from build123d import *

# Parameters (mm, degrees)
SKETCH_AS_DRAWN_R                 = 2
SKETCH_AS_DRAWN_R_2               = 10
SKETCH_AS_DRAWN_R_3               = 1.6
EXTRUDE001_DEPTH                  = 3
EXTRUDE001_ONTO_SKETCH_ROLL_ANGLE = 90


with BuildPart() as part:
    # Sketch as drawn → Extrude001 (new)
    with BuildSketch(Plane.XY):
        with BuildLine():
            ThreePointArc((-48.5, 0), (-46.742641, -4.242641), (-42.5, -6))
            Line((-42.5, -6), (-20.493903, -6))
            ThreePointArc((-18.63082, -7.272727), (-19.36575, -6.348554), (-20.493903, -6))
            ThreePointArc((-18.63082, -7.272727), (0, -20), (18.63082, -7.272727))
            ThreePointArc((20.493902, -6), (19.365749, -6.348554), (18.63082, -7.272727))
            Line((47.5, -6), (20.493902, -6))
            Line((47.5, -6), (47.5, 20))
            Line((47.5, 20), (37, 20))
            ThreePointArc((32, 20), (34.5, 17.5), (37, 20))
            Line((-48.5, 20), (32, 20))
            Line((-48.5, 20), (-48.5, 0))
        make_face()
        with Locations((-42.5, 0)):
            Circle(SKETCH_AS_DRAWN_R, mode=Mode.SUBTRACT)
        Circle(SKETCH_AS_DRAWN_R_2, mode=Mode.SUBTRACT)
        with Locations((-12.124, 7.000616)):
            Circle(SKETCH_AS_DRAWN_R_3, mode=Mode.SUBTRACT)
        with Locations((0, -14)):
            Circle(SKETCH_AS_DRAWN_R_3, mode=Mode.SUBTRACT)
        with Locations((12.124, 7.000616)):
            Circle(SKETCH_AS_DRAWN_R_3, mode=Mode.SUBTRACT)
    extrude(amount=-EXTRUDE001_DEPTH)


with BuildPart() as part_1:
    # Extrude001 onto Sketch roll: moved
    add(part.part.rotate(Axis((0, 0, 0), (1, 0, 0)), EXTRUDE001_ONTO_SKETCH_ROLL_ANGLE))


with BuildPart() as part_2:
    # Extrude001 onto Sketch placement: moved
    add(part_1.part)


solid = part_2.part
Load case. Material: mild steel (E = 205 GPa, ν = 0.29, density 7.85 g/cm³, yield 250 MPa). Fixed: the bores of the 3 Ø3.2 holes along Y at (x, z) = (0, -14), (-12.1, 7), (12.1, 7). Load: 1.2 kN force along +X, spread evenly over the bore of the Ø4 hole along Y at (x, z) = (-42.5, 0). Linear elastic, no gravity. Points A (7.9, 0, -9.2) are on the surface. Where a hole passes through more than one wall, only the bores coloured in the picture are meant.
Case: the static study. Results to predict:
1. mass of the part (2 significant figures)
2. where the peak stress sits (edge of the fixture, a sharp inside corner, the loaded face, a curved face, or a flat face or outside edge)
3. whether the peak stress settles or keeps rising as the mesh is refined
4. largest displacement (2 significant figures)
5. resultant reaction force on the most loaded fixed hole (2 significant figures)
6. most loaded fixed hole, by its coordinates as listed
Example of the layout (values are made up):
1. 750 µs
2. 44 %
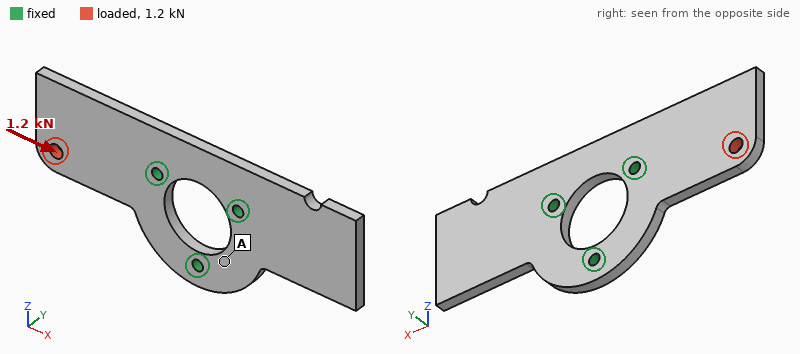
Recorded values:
1. 59 g
2. edge of the fixture
3. keeps rising
4. 10 µm
5. 820 N
6. (-12.1, 7)
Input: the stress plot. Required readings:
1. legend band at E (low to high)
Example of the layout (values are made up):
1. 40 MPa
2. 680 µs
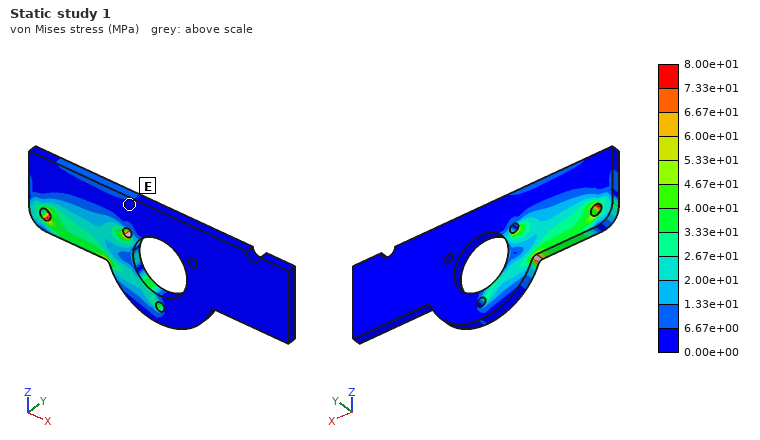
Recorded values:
1. 0.00e+00 to 6.67e+00 MPa
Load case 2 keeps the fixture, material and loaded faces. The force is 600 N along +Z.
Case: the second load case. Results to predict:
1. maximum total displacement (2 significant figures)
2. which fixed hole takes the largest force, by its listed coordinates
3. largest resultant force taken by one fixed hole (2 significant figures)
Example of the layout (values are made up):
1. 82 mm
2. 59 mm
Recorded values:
1. 19 µm
2. (0, -14)
3. 740 N
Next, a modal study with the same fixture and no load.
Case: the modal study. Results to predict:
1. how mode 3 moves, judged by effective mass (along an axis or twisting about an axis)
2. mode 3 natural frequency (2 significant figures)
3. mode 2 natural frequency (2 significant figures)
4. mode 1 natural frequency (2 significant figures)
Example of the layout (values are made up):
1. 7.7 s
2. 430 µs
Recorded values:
1. twisting about X
2. 5000 Hz
3. 1900 Hz
4. 1900 Hz
